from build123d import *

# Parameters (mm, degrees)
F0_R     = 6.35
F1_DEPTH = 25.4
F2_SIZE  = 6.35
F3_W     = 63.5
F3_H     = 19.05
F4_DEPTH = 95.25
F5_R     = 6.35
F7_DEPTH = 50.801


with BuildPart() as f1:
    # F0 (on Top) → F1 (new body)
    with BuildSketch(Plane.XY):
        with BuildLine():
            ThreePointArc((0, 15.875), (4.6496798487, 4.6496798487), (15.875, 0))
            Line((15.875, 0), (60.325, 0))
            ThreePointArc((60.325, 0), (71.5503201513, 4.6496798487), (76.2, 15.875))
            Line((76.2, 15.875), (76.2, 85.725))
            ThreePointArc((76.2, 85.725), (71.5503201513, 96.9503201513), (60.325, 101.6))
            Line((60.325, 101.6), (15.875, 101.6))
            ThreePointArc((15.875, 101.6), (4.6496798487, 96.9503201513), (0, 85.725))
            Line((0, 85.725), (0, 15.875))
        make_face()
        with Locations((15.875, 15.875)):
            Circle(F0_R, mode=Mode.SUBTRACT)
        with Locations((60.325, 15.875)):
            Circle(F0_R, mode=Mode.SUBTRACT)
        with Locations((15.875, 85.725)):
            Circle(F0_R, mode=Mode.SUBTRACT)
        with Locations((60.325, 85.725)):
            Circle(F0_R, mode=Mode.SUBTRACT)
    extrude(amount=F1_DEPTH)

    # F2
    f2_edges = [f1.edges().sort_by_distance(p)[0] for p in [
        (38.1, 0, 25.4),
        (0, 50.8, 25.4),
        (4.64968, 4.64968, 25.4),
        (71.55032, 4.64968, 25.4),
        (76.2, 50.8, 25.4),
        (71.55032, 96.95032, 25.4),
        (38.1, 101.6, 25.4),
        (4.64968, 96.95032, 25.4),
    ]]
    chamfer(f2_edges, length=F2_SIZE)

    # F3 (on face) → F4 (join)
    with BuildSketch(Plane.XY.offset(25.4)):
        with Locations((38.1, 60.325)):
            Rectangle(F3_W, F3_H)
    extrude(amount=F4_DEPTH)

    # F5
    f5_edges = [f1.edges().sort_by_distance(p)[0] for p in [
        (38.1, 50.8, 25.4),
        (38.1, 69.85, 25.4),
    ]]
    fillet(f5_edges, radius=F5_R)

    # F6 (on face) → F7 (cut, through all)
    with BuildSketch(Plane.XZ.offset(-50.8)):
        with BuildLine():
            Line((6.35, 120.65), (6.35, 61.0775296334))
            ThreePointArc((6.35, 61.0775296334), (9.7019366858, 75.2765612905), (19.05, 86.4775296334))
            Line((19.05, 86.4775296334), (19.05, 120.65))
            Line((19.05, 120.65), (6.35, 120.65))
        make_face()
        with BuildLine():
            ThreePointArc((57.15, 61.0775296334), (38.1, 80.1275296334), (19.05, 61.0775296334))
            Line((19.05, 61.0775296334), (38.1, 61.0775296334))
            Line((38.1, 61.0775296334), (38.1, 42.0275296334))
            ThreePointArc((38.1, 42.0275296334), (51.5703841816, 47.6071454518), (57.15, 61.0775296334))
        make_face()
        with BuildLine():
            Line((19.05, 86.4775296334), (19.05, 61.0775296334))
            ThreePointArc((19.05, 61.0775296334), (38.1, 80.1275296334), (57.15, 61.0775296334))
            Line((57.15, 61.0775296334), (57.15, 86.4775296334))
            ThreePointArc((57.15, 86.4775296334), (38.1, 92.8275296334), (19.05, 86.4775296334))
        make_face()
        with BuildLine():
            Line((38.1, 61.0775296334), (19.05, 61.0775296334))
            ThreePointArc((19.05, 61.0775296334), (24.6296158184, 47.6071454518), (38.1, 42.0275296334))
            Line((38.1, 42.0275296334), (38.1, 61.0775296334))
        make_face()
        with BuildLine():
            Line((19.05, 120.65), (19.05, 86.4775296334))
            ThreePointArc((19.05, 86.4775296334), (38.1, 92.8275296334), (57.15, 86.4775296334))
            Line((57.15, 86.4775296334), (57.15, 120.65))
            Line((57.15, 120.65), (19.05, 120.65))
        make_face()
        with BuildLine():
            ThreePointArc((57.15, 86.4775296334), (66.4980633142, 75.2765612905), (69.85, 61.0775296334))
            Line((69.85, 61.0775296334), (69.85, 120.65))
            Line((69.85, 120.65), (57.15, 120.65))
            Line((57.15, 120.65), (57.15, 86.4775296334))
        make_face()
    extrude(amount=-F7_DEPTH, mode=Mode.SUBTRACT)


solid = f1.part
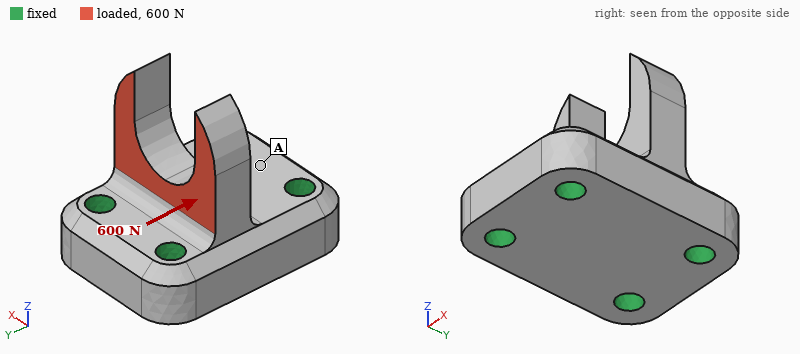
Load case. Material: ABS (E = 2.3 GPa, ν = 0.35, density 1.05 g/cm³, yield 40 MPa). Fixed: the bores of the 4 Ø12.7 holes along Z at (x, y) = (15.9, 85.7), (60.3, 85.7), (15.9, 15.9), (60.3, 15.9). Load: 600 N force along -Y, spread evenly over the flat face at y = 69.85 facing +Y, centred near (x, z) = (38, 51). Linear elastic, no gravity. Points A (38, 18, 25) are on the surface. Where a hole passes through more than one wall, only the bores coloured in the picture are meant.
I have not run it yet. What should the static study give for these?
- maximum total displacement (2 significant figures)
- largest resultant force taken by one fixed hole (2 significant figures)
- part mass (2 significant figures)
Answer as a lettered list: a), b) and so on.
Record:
a) 0.27 mm
b) 270 N
c) 220 g
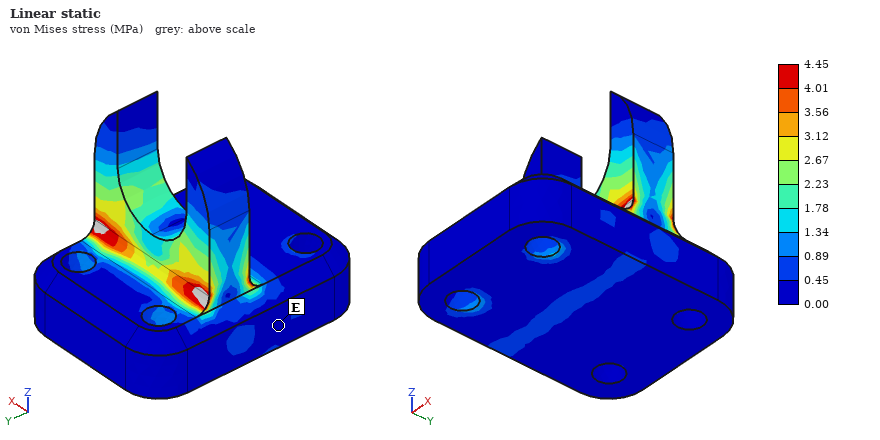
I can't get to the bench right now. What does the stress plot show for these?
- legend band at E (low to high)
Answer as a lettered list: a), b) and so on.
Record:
a) 0.00 to 0.45 MPa
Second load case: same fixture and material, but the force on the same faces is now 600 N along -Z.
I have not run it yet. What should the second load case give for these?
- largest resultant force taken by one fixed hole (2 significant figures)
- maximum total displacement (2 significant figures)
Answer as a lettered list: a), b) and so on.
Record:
a) 250 N
b) 0.13 mm
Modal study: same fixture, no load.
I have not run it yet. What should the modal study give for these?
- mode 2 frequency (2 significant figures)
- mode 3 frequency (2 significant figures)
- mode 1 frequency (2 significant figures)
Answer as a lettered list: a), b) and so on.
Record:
a) 1800 Hz
b) 1900 Hz
c) 1700 Hz
